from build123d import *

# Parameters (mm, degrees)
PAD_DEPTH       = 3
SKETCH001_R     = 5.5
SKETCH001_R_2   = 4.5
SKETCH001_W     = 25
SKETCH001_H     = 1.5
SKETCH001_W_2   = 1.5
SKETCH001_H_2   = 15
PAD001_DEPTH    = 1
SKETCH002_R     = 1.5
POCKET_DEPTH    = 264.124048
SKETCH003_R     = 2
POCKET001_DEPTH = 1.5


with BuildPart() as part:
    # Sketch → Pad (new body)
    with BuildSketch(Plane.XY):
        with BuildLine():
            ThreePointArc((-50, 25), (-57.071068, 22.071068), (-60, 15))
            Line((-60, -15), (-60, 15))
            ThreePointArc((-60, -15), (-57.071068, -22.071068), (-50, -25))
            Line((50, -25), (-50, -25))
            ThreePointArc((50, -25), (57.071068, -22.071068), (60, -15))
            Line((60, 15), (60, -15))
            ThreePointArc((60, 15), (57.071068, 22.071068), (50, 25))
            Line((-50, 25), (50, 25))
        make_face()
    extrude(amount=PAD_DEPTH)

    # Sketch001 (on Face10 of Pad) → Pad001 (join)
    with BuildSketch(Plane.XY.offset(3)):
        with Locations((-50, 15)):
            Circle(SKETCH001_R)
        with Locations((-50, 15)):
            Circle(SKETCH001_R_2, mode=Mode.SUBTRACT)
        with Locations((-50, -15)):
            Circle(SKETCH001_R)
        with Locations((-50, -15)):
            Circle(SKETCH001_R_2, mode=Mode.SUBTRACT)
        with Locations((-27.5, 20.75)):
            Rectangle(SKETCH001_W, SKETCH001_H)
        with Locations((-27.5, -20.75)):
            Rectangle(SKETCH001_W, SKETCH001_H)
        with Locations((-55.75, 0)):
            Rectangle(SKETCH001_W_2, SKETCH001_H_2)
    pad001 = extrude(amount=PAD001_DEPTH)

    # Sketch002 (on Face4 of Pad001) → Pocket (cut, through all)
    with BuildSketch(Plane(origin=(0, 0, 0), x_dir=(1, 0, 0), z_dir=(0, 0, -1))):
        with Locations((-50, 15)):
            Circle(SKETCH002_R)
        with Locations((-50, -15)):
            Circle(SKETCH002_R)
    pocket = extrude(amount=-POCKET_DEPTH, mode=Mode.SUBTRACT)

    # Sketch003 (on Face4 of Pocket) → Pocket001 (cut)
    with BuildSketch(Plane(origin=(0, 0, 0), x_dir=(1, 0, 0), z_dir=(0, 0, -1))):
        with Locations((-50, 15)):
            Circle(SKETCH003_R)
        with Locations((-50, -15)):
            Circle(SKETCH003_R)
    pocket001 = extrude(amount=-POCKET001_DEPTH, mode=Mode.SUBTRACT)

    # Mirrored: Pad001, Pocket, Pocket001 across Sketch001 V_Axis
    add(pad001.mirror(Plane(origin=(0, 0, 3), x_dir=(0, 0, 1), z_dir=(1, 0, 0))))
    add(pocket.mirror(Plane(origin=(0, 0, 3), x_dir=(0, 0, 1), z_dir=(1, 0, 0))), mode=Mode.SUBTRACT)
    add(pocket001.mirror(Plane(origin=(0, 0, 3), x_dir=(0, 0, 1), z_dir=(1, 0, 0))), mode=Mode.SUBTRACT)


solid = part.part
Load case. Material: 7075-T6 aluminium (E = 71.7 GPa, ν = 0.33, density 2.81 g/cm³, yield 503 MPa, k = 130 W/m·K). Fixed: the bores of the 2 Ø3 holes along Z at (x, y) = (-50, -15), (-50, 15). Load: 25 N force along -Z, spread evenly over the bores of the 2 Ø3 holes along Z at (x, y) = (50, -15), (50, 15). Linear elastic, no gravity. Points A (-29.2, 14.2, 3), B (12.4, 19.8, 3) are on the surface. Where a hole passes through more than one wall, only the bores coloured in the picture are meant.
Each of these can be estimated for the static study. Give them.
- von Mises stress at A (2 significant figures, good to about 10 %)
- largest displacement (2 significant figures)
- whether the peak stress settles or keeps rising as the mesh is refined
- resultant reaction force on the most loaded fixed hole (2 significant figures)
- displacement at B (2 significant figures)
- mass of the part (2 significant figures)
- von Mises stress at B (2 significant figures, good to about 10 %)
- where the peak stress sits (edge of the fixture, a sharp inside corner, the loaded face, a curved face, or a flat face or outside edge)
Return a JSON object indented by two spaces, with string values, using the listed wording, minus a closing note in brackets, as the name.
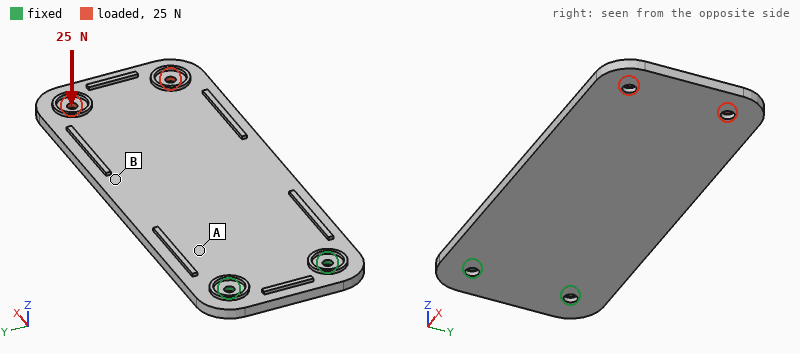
{
  "von Mises stress at A": "22 MPa",
  "largest displacement": "1.3 mm",
  "whether the peak stress settles or keeps rising as the mesh is refined": "keeps rising",
  "resultant reaction force on the most loaded fixed hole": "40 N",
  "displacement at B": "0.57 mm",
  "mass of the part": "50 g",
  "von Mises stress at B": "13 MPa",
  "where the peak stress sits": "edge of the fixture"
}
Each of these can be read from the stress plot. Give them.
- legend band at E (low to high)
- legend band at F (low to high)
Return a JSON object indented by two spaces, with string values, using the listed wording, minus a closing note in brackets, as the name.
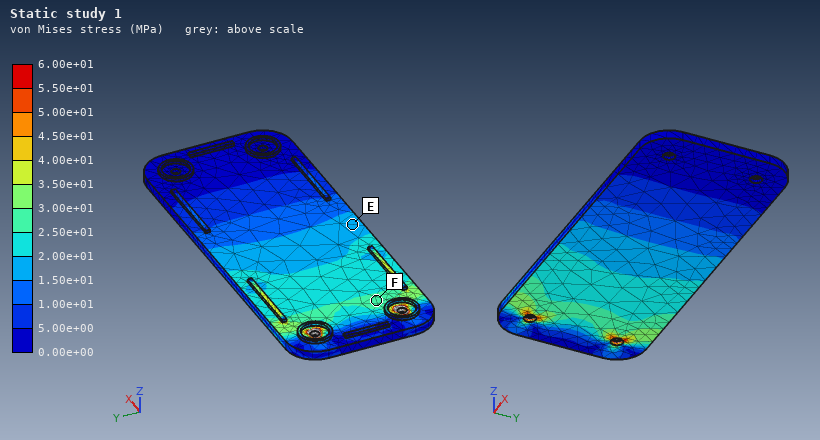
{
  "legend band at E": "1.50e+01 to 2.00e+01 MPa",
  "legend band at F": "2.50e+01 to 3.00e+01 MPa"
}
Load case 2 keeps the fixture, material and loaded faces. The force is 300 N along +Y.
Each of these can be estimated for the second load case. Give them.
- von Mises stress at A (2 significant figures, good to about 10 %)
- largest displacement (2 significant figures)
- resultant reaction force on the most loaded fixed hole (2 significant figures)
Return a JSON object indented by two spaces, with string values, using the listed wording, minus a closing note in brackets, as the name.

{
  "von Mises stress at A": "13 MPa",
  "largest displacement": "0.10 mm",
  "resultant reaction force on the most loaded fixed hole": "980 N"
}
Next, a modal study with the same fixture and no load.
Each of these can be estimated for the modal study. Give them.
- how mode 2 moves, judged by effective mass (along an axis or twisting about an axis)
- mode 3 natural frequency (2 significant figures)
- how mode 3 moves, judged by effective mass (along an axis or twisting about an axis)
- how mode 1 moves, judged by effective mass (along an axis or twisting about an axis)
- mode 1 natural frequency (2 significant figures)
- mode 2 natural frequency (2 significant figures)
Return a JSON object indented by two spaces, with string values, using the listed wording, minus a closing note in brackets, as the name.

{
  "how mode 2 moves, judged by effective mass": "twisting about X",
  "mode 3 natural frequency": "1200 Hz",
  "how mode 3 moves, judged by effective mass": "along Z",
  "how mode 1 moves, judged by effective mass": "along Z",
  "mode 1 natural frequency": "190 Hz",
  "mode 2 natural frequency": "920 Hz"
}
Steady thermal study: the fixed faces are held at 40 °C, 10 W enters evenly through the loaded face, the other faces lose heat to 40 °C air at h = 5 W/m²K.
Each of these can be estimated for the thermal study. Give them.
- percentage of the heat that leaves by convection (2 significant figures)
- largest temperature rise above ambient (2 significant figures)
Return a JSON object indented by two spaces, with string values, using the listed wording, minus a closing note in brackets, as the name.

{
  "percentage of the heat that leaves by convection": "16 %",
  "largest temperature rise above ambient": "52 K"
}
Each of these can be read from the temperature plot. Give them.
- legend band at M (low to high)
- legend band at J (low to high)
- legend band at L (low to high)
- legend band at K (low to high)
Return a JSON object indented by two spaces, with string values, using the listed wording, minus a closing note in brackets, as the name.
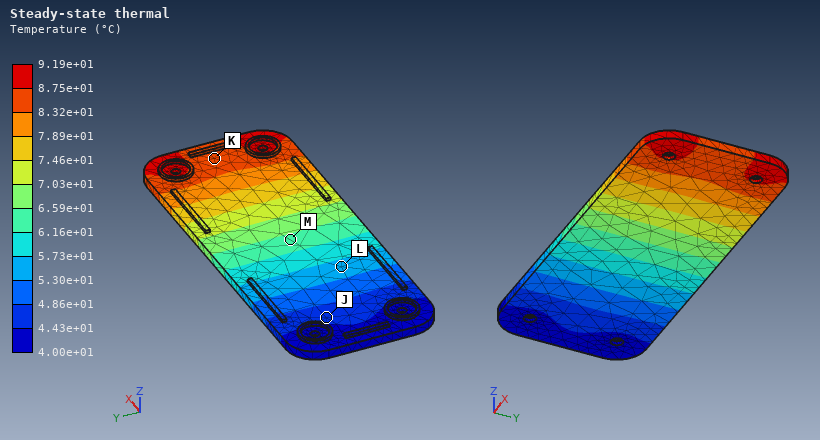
{
  "legend band at M": "6.16e+01 to 6.59e+01 °C",
  "legend band at J": "4.43e+01 to 4.86e+01 °C",
  "legend band at L": "5.30e+01 to 5.73e+01 °C",
  "legend band at K": "8.32e+01 to 8.75e+01 °C"
}
